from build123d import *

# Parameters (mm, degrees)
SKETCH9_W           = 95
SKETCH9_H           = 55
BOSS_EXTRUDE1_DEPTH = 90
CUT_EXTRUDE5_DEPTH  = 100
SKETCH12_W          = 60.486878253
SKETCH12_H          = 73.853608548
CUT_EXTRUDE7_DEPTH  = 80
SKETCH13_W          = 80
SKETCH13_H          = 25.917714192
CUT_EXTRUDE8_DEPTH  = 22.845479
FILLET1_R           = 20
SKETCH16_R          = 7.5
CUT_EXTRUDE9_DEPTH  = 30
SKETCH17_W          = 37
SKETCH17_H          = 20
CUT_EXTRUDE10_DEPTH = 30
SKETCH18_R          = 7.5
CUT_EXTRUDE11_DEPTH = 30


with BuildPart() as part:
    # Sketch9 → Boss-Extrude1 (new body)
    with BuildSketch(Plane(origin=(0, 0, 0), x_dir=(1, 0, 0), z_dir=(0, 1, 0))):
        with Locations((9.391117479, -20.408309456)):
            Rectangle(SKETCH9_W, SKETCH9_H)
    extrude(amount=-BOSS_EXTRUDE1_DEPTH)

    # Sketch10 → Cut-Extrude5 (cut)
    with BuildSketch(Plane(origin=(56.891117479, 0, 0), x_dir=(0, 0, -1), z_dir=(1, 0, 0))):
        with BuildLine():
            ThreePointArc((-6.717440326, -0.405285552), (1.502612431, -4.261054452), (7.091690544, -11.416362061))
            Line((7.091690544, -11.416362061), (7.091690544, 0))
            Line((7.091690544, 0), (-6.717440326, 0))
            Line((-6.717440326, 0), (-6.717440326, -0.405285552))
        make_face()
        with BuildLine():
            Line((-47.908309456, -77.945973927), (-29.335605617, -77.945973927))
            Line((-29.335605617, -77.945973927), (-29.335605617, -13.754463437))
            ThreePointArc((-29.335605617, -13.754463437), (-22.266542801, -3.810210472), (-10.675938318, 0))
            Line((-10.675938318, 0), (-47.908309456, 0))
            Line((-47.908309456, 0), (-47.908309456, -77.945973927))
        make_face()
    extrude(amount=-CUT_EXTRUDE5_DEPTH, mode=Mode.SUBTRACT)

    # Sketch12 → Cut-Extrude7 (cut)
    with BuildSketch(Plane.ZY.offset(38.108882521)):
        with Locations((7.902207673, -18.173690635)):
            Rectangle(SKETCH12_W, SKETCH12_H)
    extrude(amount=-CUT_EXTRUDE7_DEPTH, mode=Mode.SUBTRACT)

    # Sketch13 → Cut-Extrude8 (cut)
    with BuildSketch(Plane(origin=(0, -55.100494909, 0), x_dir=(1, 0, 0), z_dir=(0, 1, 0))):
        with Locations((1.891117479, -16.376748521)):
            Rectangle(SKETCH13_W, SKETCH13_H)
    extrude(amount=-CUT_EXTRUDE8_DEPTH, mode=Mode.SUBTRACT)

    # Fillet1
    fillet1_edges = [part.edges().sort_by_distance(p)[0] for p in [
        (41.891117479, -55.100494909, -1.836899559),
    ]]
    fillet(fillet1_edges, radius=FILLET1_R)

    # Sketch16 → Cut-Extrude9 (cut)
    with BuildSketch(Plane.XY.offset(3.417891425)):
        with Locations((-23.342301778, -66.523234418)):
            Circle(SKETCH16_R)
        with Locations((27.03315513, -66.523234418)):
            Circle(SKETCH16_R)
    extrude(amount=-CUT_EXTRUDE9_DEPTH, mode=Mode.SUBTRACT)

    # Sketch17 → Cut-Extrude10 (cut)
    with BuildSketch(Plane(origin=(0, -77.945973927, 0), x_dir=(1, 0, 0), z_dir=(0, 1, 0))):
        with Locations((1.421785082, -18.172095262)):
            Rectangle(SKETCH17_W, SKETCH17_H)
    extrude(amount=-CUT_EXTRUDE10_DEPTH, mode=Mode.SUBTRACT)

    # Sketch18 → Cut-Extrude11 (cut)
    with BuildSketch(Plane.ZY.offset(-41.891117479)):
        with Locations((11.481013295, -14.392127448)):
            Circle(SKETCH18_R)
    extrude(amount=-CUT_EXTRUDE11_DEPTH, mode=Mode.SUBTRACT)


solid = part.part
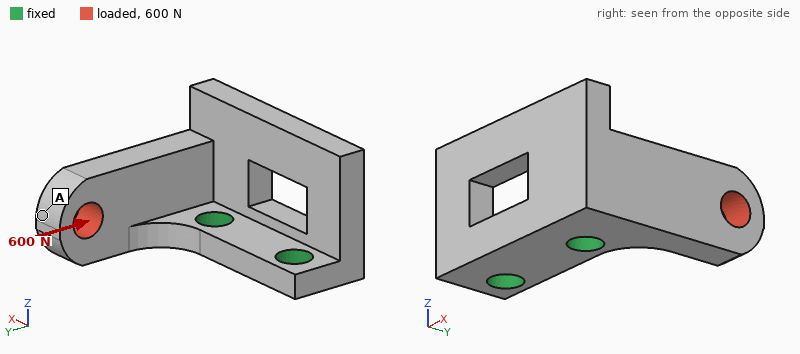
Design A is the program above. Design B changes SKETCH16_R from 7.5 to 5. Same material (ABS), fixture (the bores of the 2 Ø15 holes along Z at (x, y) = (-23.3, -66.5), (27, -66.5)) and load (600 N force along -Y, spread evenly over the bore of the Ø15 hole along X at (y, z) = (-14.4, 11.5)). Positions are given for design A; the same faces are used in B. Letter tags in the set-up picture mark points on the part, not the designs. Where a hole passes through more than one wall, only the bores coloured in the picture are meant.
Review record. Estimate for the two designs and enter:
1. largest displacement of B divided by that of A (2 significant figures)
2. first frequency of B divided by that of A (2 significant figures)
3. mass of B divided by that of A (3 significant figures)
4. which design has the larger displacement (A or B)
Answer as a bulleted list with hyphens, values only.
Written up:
- 1.4
- 0.86
- 1.02
- B
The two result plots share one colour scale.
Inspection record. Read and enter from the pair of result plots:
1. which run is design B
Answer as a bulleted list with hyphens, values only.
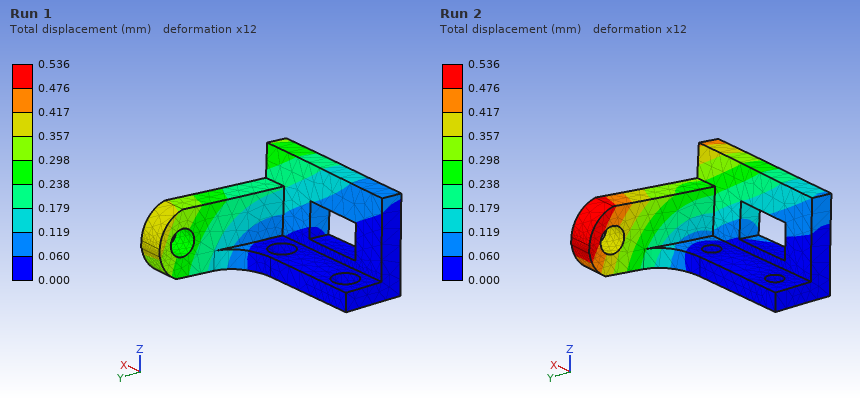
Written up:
- Run 2
